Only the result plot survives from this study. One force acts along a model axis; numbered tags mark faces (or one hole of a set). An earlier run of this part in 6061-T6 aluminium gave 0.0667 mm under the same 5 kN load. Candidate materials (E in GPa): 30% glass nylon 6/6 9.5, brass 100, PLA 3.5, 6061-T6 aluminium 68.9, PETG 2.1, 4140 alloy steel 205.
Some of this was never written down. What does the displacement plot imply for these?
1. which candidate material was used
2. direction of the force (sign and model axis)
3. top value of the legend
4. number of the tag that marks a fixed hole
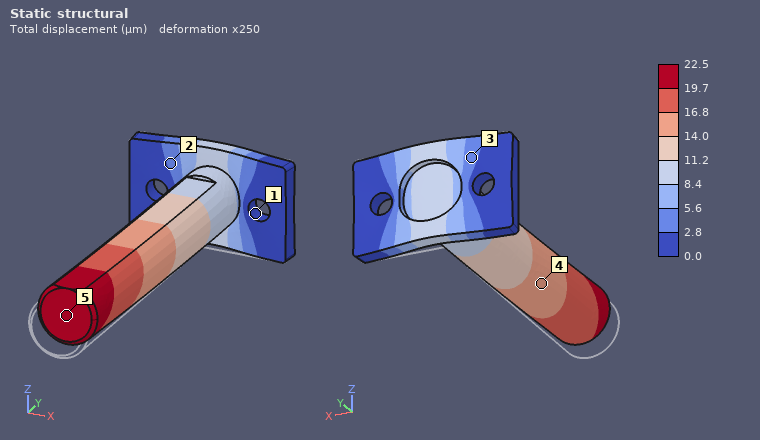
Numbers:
4140 alloy steel
+Y
22.5 µm
1
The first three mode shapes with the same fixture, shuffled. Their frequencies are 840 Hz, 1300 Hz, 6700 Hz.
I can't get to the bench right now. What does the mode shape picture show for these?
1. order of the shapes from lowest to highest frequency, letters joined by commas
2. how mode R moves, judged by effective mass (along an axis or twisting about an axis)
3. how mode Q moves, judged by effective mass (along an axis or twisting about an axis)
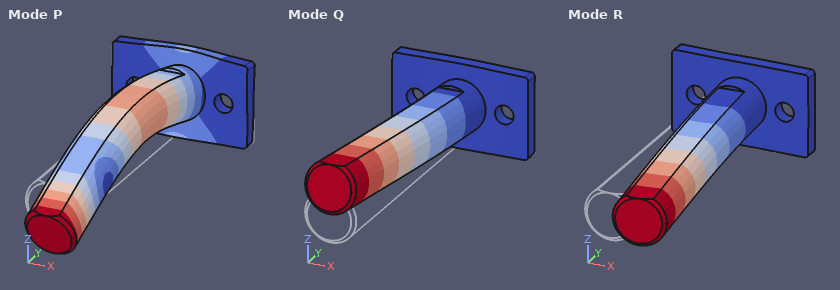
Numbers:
Q, R, P
along X
along Z
